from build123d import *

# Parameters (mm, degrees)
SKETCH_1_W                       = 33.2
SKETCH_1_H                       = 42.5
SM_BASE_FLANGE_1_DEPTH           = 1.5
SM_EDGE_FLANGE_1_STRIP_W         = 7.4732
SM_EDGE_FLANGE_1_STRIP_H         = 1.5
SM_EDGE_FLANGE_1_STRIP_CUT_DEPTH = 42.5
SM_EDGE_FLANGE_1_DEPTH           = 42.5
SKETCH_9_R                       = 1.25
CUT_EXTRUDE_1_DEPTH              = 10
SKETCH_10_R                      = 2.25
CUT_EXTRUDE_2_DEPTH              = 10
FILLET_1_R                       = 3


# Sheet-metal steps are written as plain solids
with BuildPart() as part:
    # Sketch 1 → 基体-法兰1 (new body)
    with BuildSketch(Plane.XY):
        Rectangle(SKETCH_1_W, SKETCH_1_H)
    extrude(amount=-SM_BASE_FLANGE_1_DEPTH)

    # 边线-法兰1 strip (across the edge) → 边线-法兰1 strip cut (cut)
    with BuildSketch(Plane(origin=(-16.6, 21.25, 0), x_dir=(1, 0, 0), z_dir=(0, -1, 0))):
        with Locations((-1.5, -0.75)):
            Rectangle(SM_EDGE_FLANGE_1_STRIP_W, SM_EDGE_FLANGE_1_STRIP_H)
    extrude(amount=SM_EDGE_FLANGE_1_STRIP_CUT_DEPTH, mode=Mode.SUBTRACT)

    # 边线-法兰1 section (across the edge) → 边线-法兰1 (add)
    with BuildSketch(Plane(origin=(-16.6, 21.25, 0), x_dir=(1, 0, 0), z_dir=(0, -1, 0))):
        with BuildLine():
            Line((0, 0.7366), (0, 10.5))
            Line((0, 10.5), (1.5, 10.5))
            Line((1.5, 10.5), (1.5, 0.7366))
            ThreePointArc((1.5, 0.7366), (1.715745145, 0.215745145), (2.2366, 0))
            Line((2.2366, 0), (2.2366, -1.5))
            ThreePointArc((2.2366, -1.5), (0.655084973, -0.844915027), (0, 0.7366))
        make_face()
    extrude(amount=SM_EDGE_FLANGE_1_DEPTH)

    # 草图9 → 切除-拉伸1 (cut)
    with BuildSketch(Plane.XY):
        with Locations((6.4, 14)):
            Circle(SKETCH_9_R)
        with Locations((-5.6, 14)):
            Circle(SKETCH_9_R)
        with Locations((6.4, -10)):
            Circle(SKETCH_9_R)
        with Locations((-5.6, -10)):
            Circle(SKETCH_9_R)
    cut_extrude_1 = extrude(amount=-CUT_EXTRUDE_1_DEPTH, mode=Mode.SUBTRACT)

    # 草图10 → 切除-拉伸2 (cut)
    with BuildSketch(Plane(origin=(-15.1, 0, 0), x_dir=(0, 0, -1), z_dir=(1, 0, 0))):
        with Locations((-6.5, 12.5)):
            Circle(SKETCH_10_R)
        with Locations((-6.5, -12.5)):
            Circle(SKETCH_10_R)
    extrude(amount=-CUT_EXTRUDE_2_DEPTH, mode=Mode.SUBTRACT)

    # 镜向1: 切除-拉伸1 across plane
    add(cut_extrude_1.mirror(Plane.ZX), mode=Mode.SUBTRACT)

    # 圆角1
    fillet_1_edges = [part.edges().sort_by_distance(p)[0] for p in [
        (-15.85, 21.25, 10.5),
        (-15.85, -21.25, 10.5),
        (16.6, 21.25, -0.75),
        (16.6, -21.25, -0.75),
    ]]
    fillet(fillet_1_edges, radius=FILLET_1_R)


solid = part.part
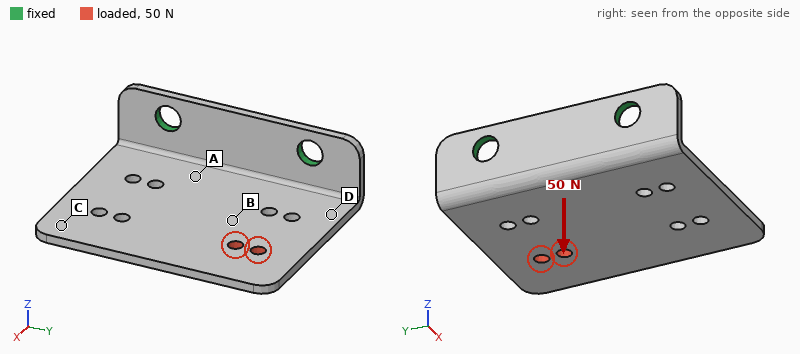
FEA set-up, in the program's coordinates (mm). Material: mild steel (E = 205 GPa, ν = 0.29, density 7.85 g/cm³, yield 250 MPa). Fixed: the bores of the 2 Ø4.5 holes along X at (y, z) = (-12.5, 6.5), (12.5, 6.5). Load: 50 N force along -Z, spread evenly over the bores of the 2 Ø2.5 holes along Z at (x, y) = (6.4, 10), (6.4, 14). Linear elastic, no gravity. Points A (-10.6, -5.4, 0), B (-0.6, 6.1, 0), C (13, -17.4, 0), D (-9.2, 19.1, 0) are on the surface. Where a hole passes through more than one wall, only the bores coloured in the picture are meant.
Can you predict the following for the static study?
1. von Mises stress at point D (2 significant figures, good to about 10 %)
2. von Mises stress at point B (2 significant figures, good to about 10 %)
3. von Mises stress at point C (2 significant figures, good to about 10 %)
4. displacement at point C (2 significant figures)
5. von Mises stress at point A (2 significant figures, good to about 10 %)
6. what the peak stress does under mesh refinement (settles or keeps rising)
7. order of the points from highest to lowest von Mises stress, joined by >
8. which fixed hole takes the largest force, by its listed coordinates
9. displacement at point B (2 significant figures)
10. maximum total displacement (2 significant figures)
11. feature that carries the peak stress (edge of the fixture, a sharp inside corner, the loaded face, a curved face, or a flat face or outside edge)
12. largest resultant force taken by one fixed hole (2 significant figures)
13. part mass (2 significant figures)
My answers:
64 MPa
36 MPa
9.5 MPa
0.14 mm
50 MPa
keeps rising
D > A > B > C
(12.5, 6.5)
0.090 mm
0.26 mm
edge of the fixture
46 N
21 g
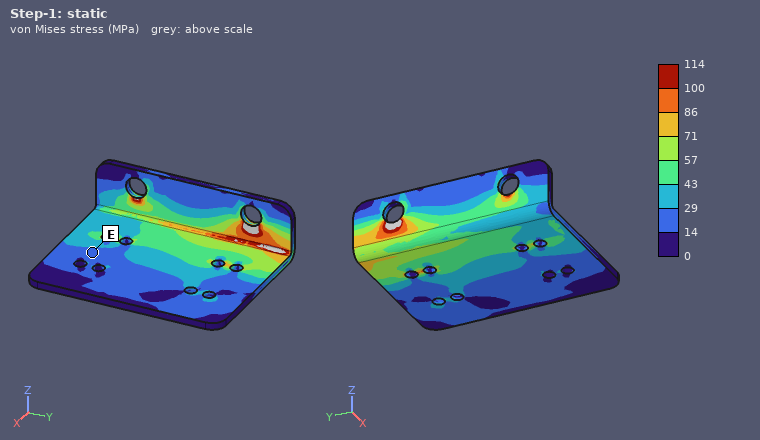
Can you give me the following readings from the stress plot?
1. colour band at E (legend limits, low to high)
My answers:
14 to 29 MPa
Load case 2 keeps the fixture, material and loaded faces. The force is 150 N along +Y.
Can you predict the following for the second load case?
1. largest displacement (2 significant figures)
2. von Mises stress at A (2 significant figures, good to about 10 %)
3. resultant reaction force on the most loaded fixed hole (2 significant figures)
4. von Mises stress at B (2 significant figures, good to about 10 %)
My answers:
32 µm
22 MPa
150 N
11 MPa
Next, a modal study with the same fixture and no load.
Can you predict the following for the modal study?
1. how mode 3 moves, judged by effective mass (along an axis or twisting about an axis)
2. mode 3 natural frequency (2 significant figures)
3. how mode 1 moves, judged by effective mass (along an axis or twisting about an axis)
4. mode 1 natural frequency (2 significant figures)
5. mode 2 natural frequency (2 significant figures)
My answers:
along Y
4500 Hz
along Z
910 Hz
2100 Hz
